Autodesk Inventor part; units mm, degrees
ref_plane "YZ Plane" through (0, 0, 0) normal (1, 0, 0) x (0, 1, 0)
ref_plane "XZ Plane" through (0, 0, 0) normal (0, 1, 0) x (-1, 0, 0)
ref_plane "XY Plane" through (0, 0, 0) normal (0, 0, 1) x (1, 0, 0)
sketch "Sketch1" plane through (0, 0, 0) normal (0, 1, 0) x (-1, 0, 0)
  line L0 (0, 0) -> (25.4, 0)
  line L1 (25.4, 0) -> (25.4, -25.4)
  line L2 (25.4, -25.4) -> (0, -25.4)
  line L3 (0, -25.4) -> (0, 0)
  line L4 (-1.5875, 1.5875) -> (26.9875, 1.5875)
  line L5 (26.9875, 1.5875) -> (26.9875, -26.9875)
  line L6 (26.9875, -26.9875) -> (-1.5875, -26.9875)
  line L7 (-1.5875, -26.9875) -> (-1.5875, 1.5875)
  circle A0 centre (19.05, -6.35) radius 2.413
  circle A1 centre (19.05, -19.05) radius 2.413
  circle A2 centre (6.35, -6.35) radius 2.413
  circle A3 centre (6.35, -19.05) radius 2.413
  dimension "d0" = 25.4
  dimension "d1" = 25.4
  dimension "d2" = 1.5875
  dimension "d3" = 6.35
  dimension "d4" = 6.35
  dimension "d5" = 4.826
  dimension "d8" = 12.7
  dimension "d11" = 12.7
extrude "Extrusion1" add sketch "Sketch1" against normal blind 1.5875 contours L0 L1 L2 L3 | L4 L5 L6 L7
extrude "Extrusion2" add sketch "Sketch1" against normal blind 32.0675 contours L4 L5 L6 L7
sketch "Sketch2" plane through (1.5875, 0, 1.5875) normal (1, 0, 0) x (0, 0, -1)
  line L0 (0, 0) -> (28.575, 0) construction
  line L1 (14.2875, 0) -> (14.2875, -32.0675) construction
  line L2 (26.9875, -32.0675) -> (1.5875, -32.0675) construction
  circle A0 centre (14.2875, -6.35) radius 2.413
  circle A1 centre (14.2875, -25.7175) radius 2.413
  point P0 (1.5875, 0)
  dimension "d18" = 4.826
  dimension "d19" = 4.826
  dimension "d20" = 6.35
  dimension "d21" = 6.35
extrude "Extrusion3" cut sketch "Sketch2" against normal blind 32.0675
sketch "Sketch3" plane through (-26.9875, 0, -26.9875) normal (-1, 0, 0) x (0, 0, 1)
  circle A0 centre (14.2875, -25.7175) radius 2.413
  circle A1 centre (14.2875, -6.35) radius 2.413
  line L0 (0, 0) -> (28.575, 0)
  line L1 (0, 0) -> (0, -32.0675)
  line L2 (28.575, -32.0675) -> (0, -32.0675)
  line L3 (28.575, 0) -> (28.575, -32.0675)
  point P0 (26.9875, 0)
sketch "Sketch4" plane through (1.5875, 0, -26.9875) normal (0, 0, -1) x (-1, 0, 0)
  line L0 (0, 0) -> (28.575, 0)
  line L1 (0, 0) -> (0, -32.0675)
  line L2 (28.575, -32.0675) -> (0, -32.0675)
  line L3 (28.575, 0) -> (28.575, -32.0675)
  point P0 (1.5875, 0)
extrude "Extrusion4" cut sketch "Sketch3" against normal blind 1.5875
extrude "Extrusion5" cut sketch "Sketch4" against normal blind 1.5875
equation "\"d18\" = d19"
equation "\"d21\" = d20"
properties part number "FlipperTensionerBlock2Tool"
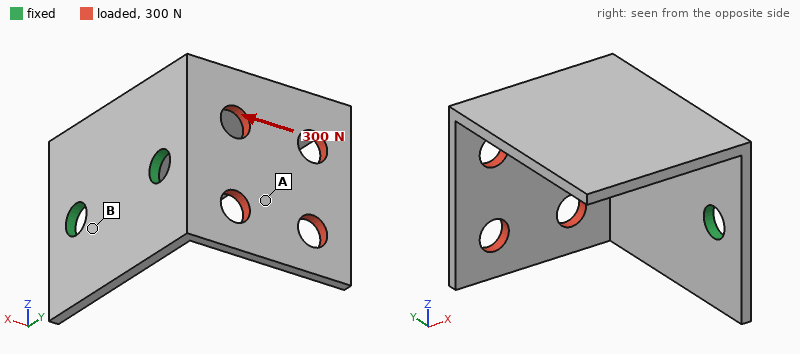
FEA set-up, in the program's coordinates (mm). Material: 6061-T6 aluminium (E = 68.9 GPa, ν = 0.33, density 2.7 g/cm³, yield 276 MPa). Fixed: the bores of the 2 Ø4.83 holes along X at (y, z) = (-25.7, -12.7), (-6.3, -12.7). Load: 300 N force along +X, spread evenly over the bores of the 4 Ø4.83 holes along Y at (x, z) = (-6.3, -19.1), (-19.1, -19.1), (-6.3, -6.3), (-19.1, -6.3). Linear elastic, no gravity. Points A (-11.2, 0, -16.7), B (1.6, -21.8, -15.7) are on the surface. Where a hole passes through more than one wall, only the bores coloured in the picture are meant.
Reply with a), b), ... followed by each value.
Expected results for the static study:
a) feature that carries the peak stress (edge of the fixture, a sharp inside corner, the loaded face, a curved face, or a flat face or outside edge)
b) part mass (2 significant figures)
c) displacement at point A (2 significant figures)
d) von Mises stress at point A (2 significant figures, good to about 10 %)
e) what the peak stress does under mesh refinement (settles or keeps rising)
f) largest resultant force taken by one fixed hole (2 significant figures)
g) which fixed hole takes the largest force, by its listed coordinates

a) edge of the fixture
b) 9.5 g
c) 41 µm
d) 15 MPa
e) keeps rising
f) 320 N
g) (-6.3, -12.7)
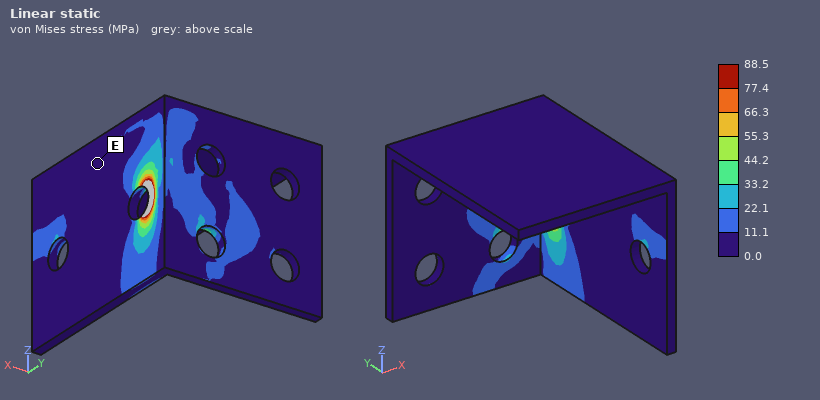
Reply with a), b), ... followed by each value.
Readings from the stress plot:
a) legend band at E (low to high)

a) 0.0 to 11.1 MPa
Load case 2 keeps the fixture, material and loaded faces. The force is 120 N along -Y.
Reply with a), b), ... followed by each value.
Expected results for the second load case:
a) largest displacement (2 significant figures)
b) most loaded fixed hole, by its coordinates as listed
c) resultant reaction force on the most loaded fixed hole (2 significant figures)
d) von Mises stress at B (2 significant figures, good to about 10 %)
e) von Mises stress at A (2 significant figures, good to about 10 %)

a) 0.34 mm
b) (-6.3, -12.7)
c) 96 N
d) 8.8 MPa
e) 32 MPa
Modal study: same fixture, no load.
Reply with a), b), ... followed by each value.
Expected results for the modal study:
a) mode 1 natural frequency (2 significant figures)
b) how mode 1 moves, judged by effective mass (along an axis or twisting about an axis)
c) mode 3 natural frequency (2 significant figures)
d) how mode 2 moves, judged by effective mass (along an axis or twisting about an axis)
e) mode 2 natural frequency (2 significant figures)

a) 1800 Hz
b) along Z
c) 3500 Hz
d) along Y
e) 2300 Hz
